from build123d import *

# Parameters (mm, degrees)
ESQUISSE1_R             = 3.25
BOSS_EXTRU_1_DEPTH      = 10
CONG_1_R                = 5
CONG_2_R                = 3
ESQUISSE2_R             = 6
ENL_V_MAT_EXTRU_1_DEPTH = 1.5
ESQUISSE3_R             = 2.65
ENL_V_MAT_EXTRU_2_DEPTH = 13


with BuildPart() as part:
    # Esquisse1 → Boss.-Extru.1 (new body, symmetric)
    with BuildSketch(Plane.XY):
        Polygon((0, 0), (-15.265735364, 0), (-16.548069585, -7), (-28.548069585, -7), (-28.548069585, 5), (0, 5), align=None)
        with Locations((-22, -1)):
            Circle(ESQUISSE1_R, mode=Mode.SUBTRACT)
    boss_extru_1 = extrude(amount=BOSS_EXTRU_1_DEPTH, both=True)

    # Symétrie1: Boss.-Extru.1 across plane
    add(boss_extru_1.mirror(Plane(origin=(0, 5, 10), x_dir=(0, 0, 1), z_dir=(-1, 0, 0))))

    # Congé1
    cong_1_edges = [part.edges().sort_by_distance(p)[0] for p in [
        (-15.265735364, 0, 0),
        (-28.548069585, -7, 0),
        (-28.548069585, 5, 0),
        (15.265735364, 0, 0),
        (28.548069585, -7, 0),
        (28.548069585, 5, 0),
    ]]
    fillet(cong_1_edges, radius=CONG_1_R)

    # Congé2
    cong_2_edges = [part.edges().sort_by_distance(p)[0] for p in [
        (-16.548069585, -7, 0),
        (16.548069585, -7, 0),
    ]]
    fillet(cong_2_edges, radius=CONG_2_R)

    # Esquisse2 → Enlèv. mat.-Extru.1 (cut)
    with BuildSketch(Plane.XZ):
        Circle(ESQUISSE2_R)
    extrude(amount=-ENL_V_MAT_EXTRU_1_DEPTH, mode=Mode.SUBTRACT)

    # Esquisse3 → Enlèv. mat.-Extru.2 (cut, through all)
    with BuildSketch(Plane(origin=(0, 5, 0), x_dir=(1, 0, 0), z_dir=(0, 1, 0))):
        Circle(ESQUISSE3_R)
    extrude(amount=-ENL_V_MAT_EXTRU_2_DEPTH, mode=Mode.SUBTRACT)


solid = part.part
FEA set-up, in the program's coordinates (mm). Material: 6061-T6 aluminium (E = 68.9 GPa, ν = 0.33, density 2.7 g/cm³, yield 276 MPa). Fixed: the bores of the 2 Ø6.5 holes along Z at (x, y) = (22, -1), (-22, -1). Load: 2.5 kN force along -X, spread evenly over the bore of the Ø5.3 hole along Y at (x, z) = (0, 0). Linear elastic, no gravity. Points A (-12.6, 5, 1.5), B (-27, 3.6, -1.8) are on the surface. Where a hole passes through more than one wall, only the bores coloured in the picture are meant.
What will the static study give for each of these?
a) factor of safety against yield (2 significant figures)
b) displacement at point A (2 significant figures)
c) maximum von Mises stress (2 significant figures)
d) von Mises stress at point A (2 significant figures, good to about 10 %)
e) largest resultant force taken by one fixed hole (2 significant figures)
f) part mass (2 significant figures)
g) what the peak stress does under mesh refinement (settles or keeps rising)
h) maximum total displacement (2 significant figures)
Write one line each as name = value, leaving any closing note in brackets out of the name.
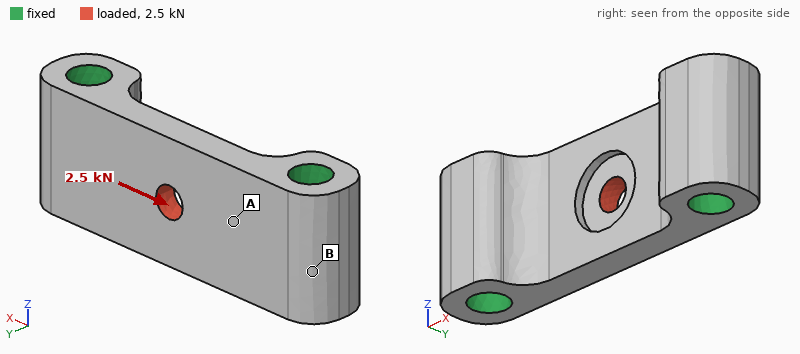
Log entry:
factor of safety against yield = 3.8
displacement at point A = 1.8 µm
maximum von Mises stress = 73 MPa
von Mises stress at point A = 14 MPa
largest resultant force taken by one fixed hole = 1.3 kN
part mass = 20 g
what the peak stress does under mesh refinement = settles
maximum total displacement = 5.9 µm
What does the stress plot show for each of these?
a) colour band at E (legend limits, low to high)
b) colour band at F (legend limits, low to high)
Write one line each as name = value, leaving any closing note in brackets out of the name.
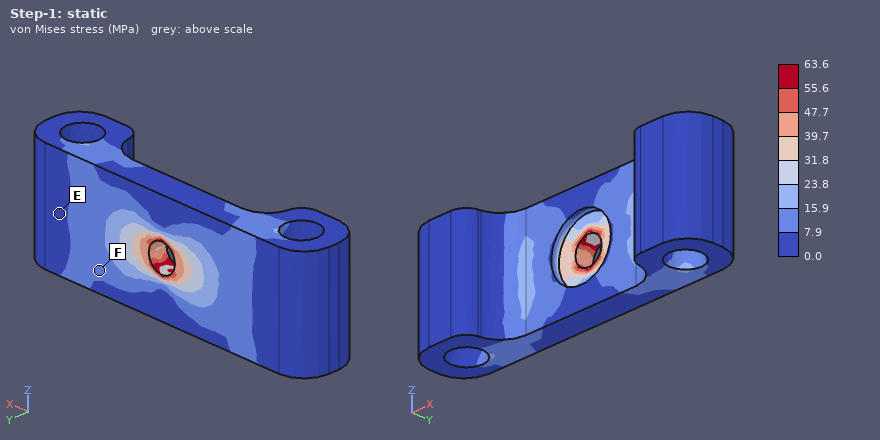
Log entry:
colour band at E = 0.0 to 7.9 MPa
colour band at F = 7.9 to 15.9 MPa
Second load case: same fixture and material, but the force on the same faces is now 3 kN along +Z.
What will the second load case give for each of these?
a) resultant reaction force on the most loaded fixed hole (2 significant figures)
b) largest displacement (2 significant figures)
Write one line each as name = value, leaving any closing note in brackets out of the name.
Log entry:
resultant reaction force on the most loaded fixed hole = 1.5 kN
largest displacement = 18 µm
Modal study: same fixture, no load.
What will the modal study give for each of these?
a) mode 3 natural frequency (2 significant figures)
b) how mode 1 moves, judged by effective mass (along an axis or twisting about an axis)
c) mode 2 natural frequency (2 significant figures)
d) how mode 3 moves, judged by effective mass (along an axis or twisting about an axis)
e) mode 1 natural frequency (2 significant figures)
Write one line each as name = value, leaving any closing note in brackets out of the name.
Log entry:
mode 3 natural frequency = 37 kHz
how mode 1 moves, judged by effective mass = along Y
mode 2 natural frequency = 28 kHz
how mode 3 moves, judged by effective mass = along Z
mode 1 natural frequency = 22 kHz
